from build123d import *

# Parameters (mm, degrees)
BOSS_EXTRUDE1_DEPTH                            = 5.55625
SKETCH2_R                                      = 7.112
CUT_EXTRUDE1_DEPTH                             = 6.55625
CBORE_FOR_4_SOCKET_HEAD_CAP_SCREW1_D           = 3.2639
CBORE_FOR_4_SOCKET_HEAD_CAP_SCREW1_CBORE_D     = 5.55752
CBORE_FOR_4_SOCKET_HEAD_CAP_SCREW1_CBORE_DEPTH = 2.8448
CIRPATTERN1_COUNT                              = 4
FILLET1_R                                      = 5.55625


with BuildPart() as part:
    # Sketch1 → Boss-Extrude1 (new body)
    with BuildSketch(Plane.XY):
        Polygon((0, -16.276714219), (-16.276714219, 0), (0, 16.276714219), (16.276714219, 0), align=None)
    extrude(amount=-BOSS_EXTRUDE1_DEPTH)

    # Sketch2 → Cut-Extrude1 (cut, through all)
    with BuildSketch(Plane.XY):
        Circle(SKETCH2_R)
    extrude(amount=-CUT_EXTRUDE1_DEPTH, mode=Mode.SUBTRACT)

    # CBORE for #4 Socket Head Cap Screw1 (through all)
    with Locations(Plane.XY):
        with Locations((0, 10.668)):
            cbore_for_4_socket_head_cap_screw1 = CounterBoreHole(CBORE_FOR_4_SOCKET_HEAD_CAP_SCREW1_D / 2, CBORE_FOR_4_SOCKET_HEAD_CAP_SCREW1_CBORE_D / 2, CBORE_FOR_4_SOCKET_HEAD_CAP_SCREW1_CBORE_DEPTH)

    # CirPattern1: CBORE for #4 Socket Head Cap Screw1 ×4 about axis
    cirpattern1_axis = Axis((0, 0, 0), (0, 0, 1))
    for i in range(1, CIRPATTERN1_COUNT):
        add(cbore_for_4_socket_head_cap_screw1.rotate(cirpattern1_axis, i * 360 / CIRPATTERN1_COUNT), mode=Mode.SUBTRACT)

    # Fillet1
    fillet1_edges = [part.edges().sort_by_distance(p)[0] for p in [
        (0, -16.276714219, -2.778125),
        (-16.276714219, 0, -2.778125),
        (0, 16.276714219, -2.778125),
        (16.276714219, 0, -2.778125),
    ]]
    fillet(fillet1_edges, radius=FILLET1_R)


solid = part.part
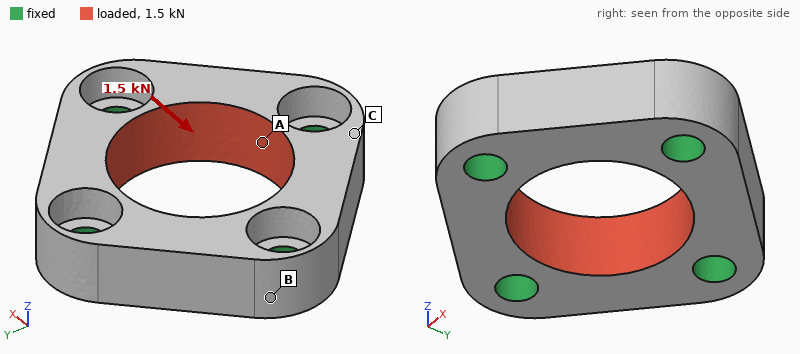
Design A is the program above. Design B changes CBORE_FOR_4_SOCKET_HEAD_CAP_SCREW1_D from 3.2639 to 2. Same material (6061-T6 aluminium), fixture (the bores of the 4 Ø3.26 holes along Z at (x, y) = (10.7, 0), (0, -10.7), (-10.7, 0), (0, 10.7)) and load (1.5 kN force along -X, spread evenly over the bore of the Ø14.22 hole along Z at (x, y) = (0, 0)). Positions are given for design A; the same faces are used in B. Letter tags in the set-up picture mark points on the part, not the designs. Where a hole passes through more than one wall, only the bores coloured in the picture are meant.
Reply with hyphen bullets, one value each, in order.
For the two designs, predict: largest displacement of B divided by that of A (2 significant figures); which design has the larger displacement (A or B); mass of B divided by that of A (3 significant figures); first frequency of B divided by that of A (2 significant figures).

- 1.2
- B
- 1.04
- 0.78
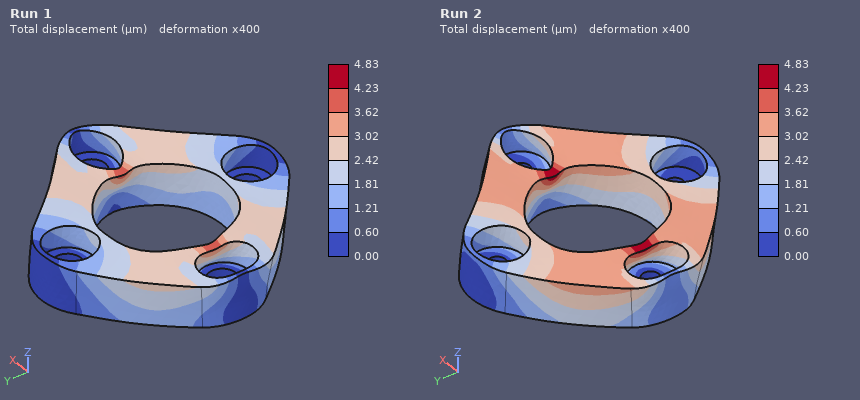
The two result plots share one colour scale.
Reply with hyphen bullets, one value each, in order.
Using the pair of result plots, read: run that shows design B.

- Run 2
